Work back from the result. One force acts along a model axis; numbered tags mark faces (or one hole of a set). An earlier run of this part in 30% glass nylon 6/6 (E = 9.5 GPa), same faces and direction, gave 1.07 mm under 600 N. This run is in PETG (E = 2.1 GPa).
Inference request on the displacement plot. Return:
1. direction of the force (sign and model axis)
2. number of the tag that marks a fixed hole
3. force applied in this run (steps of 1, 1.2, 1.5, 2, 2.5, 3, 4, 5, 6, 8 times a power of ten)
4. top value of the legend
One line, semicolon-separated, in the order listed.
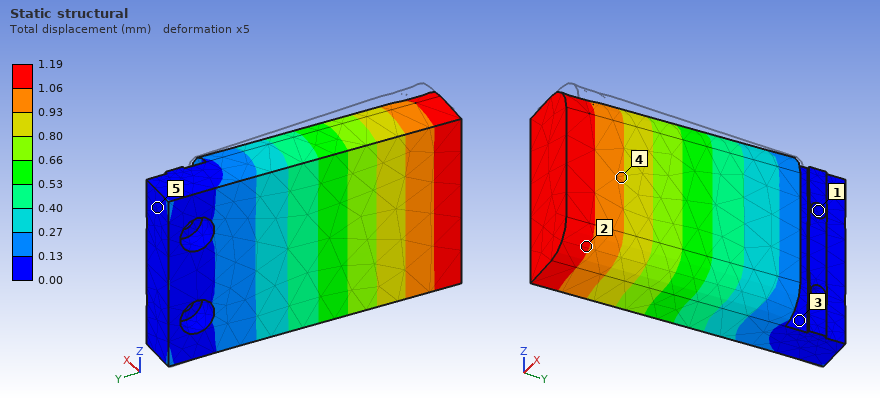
-X; 1; 150 N; 1.19 mm
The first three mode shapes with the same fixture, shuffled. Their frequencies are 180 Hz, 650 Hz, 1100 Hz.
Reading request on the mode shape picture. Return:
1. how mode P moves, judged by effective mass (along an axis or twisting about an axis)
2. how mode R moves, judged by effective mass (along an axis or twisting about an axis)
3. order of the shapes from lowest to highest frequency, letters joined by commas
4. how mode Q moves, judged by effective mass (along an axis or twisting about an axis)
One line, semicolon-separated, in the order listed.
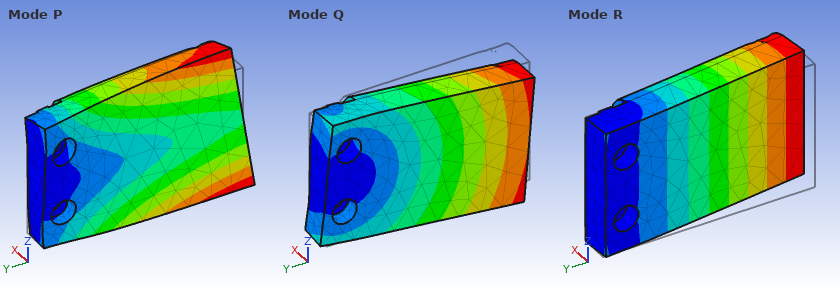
twisting about Y; along X; R, Q, P; along Z
